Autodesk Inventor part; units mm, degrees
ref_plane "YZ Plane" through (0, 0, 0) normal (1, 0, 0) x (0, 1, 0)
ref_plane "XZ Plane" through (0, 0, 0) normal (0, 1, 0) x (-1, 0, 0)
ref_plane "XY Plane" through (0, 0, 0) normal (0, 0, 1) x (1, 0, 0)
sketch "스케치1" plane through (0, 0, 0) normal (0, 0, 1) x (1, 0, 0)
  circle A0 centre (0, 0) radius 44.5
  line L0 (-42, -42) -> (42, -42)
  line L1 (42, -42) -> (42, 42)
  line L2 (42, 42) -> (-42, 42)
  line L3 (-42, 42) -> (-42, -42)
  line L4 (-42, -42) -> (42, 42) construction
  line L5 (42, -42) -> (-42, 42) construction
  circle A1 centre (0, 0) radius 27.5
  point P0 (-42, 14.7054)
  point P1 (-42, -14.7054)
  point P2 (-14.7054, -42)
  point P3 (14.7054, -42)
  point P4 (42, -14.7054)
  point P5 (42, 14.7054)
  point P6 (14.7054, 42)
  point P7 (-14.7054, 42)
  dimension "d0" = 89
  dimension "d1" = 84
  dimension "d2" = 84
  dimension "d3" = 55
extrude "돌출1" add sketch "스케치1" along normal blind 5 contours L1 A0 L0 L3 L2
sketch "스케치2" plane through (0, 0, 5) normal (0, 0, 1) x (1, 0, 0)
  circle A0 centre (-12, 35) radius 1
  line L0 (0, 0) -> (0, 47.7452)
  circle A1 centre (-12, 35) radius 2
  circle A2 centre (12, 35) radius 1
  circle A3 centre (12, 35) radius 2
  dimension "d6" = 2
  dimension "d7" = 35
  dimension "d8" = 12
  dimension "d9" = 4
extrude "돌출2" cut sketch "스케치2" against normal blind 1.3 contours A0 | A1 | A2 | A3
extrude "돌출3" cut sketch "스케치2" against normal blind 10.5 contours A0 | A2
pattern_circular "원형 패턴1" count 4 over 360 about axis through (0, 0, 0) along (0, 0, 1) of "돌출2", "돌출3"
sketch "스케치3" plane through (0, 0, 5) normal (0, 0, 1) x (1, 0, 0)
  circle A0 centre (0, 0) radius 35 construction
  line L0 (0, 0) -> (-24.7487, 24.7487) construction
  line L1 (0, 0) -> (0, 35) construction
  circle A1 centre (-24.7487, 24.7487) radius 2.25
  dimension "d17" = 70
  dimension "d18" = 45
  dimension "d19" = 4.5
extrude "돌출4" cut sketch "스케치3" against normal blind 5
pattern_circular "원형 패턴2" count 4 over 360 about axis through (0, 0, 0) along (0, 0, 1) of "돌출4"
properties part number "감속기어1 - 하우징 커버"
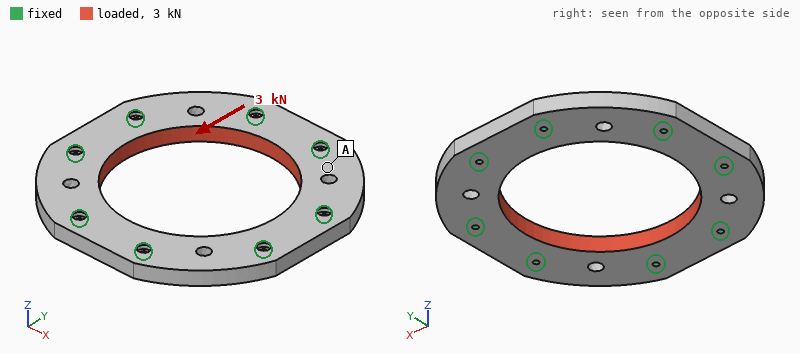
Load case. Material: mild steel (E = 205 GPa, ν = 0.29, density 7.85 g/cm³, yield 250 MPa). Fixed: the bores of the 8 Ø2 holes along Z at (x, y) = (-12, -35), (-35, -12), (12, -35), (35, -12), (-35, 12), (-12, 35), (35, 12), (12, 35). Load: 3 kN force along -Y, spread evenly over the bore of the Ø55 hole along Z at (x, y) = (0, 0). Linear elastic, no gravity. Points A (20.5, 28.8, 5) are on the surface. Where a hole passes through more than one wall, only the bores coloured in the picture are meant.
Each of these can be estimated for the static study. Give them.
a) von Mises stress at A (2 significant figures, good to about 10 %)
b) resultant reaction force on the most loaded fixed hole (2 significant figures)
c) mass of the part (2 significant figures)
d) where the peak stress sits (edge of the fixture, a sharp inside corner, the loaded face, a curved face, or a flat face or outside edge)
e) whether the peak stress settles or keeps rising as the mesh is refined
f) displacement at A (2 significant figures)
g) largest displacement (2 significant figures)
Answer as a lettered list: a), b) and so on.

a) 3.6 MPa
b) 410 N
c) 140 g
d) edge of the fixture
e) keeps rising
f) 0.55 µm
g) 0.78 µm
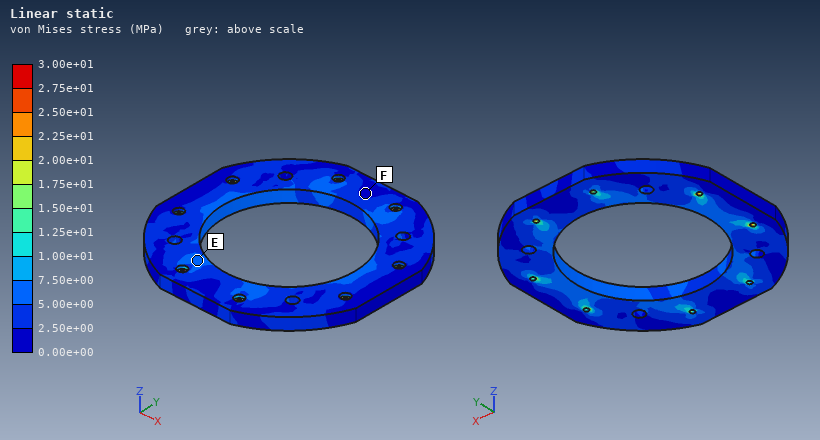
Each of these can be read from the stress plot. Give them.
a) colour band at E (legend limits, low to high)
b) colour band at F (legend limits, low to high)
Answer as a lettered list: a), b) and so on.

a) 5.00e+00 to 7.50e+00 MPa
b) 0.00e+00 to 2.50e+00 MPa
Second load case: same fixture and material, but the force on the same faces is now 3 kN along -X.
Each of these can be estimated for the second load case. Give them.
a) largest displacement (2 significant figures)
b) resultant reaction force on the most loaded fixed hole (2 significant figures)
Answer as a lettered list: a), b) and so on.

a) 0.78 µm
b) 410 N
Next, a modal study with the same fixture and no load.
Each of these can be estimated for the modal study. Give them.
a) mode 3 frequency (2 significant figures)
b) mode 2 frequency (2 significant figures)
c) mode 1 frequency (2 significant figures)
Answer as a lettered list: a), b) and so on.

a) 15 kHz
b) 15 kHz
c) 14 kHz
